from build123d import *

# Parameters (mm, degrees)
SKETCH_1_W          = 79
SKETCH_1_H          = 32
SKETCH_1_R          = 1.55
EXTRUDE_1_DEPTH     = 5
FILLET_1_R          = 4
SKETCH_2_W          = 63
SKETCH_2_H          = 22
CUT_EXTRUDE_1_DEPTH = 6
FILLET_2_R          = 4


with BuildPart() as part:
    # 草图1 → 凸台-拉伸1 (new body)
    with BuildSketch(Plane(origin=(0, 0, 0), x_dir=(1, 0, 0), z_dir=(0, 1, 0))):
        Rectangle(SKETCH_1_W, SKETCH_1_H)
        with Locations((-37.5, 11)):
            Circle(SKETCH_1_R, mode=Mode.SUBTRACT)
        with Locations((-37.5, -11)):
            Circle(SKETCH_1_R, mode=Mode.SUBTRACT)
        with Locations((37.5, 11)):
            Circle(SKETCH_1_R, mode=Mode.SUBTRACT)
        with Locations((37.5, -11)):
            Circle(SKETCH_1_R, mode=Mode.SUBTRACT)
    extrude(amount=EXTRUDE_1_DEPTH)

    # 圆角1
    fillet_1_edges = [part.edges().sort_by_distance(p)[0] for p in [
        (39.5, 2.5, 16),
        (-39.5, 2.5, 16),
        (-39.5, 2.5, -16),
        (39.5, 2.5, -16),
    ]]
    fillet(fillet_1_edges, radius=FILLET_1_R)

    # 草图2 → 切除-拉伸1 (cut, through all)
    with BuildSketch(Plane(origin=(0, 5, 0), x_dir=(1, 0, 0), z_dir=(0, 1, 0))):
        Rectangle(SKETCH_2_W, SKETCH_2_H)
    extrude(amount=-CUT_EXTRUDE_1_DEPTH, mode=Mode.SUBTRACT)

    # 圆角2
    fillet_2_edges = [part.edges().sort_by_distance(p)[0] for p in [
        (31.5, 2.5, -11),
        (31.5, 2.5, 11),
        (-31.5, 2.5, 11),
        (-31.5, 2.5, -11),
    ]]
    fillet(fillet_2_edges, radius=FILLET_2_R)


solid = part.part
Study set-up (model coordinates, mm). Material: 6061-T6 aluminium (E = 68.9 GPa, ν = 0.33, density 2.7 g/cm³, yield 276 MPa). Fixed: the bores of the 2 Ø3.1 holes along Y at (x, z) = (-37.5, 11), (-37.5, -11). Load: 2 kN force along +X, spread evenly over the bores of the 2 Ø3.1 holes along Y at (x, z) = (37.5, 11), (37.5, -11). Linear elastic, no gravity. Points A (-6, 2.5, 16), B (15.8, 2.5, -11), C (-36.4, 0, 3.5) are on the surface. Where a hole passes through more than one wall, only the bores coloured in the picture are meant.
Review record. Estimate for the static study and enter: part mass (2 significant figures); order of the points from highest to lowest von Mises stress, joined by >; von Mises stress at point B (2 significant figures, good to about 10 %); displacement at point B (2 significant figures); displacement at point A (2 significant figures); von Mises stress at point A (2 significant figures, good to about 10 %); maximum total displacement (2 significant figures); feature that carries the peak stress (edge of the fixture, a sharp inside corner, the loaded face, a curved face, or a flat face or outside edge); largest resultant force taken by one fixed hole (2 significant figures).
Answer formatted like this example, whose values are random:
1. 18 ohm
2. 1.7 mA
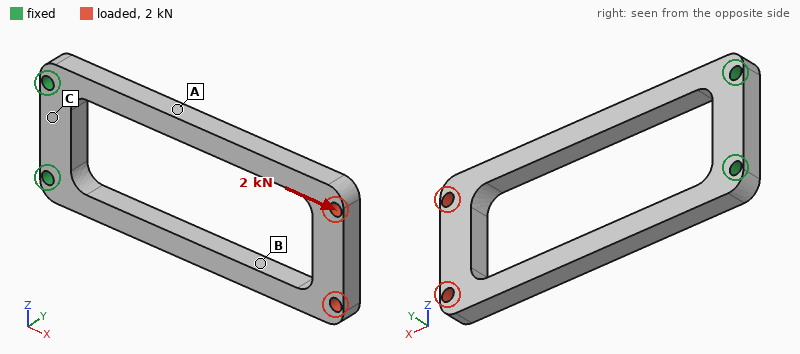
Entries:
1. 15 g
2. B > A > C
3. 56 MPa
4. 46 µm
5. 37 µm
6. 32 MPa
7. 58 µm
8. a flat face or outside edge
9. 1.0 kN
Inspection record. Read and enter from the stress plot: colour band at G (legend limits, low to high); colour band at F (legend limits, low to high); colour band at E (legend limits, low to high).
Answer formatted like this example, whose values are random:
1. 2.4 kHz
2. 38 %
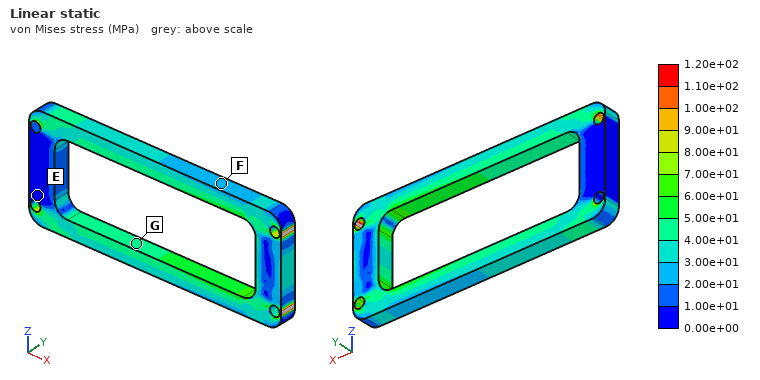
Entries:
1. 4.00e+01 to 5.00e+01 MPa
2. 2.00e+01 to 3.00e+01 MPa
3. 0.00e+00 to 1.00e+01 MPa
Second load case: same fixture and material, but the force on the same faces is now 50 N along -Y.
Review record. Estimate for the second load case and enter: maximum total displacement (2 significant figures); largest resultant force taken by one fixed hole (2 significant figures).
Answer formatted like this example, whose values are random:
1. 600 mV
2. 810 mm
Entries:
1. 0.93 mm
2. 25 N
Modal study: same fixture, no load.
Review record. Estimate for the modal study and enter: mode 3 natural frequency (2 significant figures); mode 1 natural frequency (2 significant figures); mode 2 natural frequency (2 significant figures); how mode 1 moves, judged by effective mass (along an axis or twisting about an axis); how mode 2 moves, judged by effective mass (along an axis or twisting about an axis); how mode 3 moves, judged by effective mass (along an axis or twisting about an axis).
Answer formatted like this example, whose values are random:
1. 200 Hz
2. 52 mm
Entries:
1. 1800 Hz
2. 560 Hz
3. 1100 Hz
4. along Y
5. along Z
6. twisting about X
